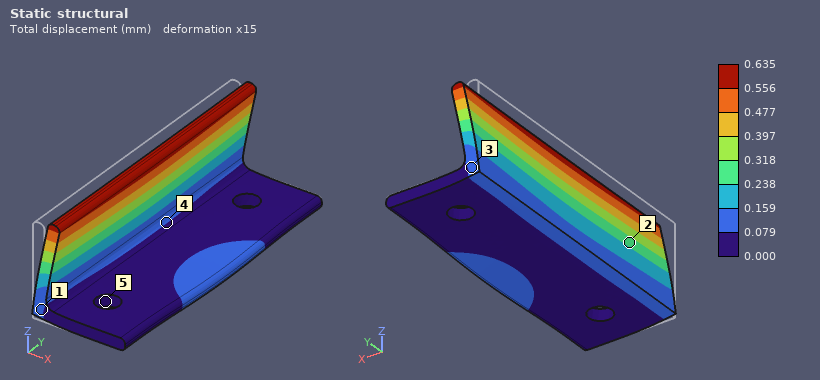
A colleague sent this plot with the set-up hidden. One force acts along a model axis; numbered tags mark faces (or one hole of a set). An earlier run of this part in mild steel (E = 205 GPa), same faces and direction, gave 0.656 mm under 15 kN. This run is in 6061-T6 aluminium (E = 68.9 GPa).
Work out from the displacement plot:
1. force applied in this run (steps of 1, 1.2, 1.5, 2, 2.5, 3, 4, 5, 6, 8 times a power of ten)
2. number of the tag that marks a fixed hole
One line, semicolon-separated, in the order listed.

5 kN; 5
